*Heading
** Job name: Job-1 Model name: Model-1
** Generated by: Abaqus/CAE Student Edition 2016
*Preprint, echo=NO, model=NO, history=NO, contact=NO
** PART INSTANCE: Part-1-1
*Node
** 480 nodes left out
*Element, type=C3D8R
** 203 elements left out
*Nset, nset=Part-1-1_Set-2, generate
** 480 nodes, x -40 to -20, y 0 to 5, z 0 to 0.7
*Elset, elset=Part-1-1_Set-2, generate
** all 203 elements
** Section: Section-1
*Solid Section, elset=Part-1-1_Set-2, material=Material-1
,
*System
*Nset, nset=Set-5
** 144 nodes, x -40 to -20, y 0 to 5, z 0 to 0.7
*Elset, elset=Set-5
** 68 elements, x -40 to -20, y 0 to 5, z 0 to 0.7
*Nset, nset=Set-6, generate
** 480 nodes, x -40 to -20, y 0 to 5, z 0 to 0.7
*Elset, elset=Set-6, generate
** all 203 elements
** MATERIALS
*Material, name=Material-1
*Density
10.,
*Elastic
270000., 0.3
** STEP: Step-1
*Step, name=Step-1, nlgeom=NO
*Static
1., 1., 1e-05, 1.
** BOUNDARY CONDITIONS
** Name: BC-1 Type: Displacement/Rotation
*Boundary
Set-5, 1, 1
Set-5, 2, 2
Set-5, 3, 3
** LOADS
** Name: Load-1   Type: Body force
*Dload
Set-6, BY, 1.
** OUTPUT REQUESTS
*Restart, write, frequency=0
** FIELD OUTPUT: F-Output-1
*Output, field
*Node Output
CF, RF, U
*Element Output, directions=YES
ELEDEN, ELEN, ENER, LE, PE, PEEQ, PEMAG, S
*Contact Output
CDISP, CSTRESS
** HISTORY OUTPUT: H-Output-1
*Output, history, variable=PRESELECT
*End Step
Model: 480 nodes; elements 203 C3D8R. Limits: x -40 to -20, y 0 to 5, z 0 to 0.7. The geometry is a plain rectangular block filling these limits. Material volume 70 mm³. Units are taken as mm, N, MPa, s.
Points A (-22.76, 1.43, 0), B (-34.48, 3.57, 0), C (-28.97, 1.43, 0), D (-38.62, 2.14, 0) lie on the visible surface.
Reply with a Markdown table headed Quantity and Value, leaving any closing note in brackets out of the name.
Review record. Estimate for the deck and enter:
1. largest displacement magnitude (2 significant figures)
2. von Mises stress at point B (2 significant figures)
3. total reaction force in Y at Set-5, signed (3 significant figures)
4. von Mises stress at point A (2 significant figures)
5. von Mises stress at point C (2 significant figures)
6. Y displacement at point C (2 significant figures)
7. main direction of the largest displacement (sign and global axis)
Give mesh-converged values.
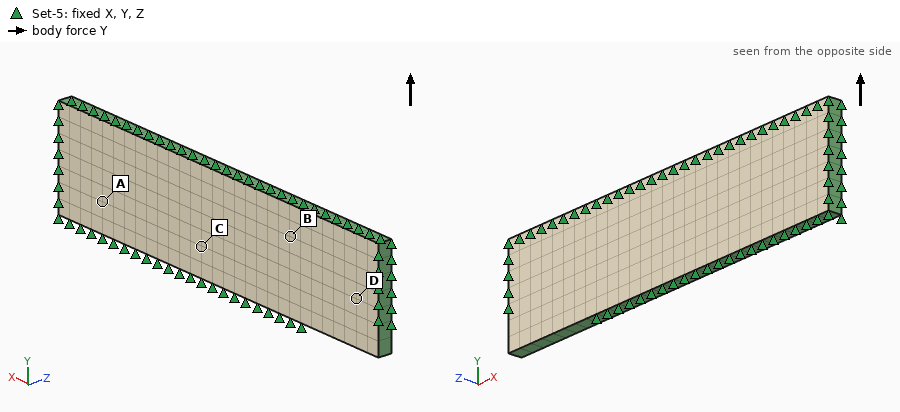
| Quantity | Value |
|---|---|
| largest displacement magnitude | 1.0e-05 mm |
| von Mises stress at point B | 0.96 MPa |
| total reaction force in Y at Set-5, signed | -70.0 N |
| von Mises stress at point A | 0.93 MPa |
| von Mises stress at point C | 0.95 MPa |
| Y displacement at point C | 8.3e-06 mm |
| main direction of the largest displacement | +Y |
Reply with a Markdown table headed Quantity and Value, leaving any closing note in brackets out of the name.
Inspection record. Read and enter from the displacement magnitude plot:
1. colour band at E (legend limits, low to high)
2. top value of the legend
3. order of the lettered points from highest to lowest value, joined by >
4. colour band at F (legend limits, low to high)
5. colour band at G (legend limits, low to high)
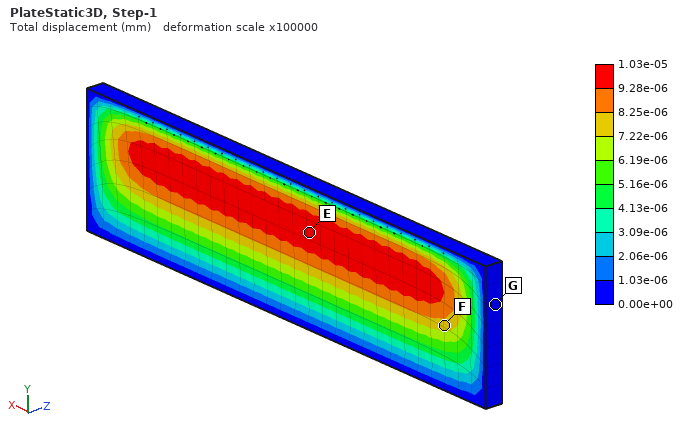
| Quantity | Value |
|---|---|
| colour band at E | 9.28e-06 to 1.03e-05 mm |
| top value of the legend | 1.03e-05 mm |
| order of the lettered points from highest to lowest value, joined by > | E > F > G |
| colour band at F | 7.22e-06 to 8.25e-06 mm |
| colour band at G | 0.00e+00 to 1.03e-06 mm |
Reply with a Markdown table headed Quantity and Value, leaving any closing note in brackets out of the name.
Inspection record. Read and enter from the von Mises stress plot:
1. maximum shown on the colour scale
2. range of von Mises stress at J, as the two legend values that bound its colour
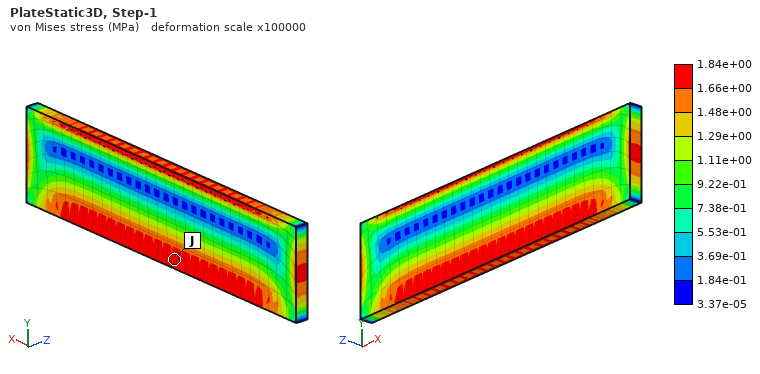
| Quantity | Value |
|---|---|
| maximum shown on the colour scale | 1.84e+00 MPa |
| range of von Mises stress at J, as the two legend values that bound its colour | 1.66e+00 to 1.84e+00 MPa |
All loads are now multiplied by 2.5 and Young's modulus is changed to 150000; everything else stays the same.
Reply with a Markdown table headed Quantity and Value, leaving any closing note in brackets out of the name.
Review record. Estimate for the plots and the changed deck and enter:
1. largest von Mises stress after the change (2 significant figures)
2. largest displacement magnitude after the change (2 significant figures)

| Quantity | Value |
|---|---|
| largest von Mises stress after the change | 4.6 MPa |
| largest displacement magnitude after the change | 4.6e-05 mm |
